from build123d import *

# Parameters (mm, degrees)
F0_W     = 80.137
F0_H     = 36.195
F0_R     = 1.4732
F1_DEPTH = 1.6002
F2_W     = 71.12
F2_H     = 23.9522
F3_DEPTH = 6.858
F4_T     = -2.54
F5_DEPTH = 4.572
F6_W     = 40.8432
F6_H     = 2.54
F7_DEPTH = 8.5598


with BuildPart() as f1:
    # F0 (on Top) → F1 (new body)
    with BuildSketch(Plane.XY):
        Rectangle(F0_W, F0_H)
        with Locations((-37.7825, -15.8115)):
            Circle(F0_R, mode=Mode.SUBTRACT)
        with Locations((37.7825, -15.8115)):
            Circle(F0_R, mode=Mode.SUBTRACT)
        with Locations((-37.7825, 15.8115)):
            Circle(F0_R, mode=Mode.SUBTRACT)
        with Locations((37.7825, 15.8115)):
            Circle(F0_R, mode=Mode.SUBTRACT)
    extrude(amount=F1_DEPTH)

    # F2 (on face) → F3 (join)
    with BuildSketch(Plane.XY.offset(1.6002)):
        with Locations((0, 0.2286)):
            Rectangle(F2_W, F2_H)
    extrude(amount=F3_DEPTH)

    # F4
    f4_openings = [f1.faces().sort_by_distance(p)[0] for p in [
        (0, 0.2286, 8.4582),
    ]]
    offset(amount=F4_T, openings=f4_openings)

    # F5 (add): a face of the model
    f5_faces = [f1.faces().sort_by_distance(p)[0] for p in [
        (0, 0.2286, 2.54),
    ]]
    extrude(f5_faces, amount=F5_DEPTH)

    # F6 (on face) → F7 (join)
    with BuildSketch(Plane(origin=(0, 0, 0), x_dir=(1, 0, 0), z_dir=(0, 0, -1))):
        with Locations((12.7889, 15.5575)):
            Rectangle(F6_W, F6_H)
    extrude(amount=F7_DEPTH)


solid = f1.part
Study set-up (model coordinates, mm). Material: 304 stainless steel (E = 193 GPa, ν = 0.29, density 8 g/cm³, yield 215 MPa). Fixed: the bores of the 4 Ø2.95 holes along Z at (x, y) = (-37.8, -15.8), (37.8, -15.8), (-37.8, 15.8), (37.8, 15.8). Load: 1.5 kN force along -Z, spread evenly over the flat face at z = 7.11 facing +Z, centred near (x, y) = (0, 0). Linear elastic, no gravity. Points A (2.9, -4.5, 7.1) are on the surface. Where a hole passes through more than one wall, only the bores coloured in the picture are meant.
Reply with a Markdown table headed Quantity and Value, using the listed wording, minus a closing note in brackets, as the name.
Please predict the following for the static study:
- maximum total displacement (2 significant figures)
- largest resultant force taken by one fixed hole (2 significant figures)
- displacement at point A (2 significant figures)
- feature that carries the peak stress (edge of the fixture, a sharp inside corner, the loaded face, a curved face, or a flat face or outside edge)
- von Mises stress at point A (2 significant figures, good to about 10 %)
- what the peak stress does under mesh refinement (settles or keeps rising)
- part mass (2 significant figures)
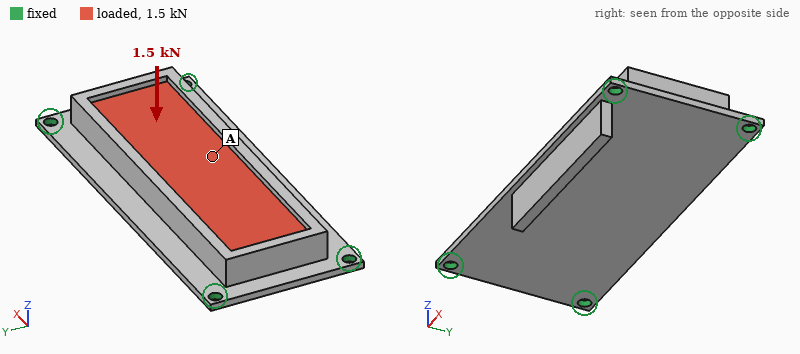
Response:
| Quantity | Value |
|---|---|
| maximum total displacement | 41 µm |
| largest resultant force taken by one fixed hole | 780 N |
| displacement at point A | 36 µm |
| feature that carries the peak stress | edge of the fixture |
| von Mises stress at point A | 38 MPa |
| what the peak stress does under mesh refinement | keeps rising |
| part mass | 120 g |
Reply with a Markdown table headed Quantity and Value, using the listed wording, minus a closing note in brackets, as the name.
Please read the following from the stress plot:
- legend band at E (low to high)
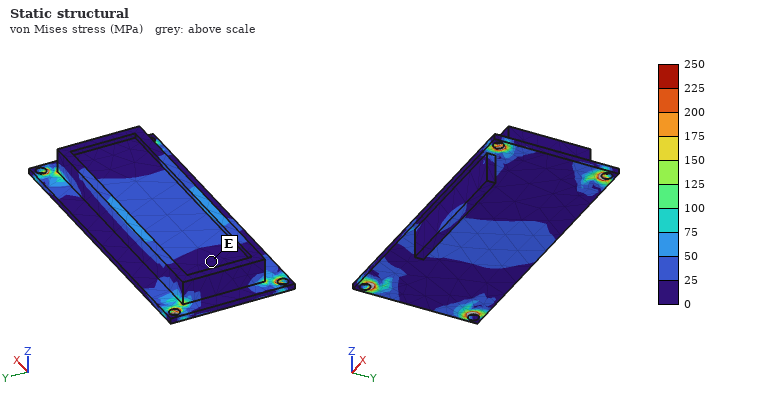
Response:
| Quantity | Value |
|---|---|
| legend band at E | 0 to 25 MPa |
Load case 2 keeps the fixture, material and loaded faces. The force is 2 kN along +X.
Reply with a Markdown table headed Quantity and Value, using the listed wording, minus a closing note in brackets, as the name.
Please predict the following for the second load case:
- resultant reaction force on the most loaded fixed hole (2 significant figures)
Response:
| Quantity | Value |
|---|---|
| resultant reaction force on the most loaded fixed hole | 570 N |
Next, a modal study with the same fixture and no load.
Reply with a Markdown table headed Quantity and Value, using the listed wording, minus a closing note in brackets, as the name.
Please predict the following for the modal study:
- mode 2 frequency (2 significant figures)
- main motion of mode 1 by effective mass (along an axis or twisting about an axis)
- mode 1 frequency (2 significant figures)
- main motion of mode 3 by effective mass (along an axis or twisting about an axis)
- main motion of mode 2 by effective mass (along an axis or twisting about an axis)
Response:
| Quantity | Value |
|---|---|
| mode 2 frequency | 5900 Hz |
| main motion of mode 1 by effective mass | along Z |
| mode 1 frequency | 3300 Hz |
| main motion of mode 3 by effective mass | twisting about Y |
| main motion of mode 2 by effective mass | twisting about X |
